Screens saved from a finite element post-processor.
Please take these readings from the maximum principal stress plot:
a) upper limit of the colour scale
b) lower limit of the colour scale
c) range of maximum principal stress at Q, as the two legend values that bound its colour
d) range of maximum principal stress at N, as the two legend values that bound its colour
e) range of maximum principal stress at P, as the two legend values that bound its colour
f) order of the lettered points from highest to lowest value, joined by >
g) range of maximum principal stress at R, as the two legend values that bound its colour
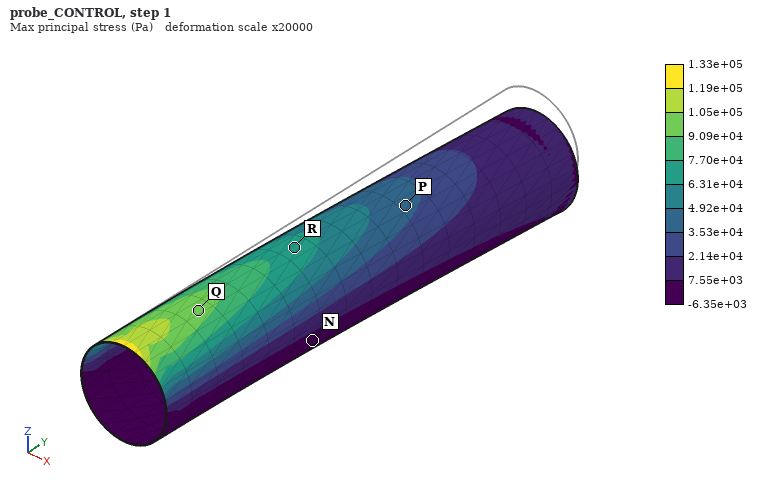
1.33e+05 Pa
-6.35e+03 Pa
9.09e+04 to 1.05e+05 Pa
-6.35e+03 to 7.55e+03 Pa
3.53e+04 to 4.92e+04 Pa
Q > R > P > N
6.31e+04 to 7.70e+04 Pa
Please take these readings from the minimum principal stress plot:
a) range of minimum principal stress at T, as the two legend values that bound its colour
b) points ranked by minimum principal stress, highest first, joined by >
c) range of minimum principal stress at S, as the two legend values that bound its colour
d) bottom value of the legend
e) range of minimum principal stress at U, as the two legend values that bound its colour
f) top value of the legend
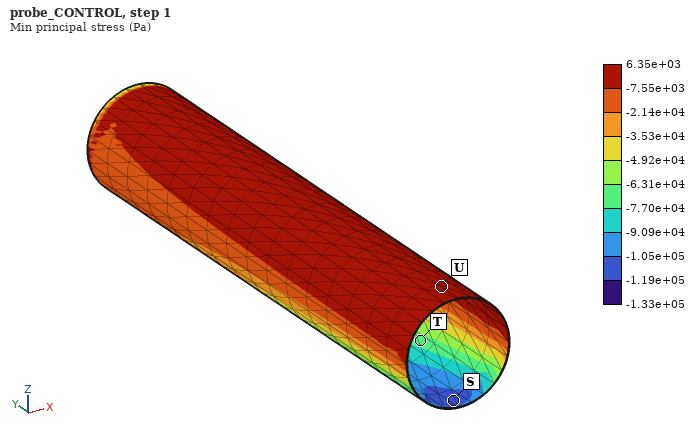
-7.70e+04 to -6.31e+04 Pa
U > T > S
-1.19e+05 to -1.05e+05 Pa
-1.33e+05 Pa
-7.55e+03 to 6.35e+03 Pa
6.35e+03 Pa
